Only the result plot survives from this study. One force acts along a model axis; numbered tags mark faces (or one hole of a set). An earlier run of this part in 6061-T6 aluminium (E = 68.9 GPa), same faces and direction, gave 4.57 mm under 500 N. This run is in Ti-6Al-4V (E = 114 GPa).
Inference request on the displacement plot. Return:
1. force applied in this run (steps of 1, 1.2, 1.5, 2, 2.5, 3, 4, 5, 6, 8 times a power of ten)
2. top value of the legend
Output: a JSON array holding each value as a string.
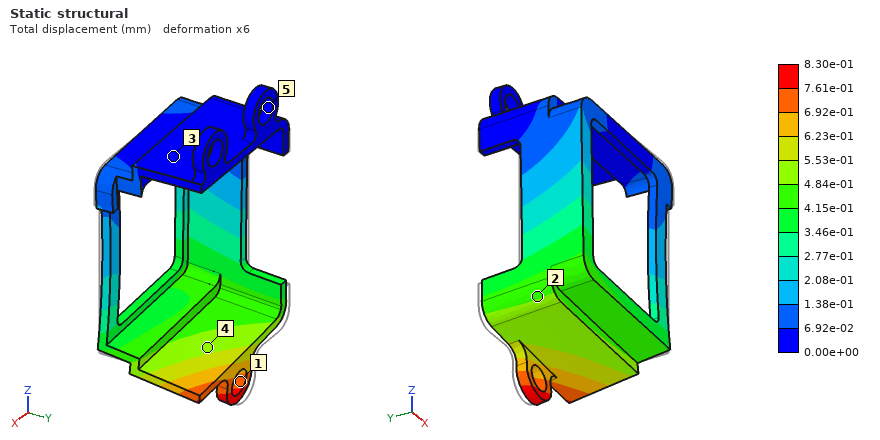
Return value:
["150 N", "8.30e-01 mm"]
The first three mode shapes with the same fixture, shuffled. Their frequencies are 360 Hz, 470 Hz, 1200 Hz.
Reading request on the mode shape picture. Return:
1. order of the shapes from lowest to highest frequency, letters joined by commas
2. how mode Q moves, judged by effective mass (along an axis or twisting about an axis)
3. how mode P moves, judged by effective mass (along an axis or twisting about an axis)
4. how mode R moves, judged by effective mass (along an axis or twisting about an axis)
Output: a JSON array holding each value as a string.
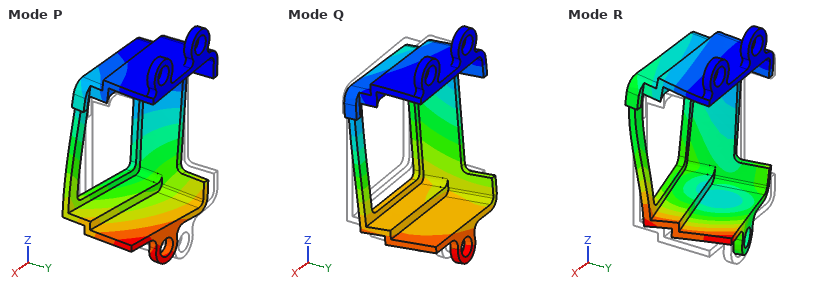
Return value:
["Q, P, R", "along Y", "along X", "along Z"]
